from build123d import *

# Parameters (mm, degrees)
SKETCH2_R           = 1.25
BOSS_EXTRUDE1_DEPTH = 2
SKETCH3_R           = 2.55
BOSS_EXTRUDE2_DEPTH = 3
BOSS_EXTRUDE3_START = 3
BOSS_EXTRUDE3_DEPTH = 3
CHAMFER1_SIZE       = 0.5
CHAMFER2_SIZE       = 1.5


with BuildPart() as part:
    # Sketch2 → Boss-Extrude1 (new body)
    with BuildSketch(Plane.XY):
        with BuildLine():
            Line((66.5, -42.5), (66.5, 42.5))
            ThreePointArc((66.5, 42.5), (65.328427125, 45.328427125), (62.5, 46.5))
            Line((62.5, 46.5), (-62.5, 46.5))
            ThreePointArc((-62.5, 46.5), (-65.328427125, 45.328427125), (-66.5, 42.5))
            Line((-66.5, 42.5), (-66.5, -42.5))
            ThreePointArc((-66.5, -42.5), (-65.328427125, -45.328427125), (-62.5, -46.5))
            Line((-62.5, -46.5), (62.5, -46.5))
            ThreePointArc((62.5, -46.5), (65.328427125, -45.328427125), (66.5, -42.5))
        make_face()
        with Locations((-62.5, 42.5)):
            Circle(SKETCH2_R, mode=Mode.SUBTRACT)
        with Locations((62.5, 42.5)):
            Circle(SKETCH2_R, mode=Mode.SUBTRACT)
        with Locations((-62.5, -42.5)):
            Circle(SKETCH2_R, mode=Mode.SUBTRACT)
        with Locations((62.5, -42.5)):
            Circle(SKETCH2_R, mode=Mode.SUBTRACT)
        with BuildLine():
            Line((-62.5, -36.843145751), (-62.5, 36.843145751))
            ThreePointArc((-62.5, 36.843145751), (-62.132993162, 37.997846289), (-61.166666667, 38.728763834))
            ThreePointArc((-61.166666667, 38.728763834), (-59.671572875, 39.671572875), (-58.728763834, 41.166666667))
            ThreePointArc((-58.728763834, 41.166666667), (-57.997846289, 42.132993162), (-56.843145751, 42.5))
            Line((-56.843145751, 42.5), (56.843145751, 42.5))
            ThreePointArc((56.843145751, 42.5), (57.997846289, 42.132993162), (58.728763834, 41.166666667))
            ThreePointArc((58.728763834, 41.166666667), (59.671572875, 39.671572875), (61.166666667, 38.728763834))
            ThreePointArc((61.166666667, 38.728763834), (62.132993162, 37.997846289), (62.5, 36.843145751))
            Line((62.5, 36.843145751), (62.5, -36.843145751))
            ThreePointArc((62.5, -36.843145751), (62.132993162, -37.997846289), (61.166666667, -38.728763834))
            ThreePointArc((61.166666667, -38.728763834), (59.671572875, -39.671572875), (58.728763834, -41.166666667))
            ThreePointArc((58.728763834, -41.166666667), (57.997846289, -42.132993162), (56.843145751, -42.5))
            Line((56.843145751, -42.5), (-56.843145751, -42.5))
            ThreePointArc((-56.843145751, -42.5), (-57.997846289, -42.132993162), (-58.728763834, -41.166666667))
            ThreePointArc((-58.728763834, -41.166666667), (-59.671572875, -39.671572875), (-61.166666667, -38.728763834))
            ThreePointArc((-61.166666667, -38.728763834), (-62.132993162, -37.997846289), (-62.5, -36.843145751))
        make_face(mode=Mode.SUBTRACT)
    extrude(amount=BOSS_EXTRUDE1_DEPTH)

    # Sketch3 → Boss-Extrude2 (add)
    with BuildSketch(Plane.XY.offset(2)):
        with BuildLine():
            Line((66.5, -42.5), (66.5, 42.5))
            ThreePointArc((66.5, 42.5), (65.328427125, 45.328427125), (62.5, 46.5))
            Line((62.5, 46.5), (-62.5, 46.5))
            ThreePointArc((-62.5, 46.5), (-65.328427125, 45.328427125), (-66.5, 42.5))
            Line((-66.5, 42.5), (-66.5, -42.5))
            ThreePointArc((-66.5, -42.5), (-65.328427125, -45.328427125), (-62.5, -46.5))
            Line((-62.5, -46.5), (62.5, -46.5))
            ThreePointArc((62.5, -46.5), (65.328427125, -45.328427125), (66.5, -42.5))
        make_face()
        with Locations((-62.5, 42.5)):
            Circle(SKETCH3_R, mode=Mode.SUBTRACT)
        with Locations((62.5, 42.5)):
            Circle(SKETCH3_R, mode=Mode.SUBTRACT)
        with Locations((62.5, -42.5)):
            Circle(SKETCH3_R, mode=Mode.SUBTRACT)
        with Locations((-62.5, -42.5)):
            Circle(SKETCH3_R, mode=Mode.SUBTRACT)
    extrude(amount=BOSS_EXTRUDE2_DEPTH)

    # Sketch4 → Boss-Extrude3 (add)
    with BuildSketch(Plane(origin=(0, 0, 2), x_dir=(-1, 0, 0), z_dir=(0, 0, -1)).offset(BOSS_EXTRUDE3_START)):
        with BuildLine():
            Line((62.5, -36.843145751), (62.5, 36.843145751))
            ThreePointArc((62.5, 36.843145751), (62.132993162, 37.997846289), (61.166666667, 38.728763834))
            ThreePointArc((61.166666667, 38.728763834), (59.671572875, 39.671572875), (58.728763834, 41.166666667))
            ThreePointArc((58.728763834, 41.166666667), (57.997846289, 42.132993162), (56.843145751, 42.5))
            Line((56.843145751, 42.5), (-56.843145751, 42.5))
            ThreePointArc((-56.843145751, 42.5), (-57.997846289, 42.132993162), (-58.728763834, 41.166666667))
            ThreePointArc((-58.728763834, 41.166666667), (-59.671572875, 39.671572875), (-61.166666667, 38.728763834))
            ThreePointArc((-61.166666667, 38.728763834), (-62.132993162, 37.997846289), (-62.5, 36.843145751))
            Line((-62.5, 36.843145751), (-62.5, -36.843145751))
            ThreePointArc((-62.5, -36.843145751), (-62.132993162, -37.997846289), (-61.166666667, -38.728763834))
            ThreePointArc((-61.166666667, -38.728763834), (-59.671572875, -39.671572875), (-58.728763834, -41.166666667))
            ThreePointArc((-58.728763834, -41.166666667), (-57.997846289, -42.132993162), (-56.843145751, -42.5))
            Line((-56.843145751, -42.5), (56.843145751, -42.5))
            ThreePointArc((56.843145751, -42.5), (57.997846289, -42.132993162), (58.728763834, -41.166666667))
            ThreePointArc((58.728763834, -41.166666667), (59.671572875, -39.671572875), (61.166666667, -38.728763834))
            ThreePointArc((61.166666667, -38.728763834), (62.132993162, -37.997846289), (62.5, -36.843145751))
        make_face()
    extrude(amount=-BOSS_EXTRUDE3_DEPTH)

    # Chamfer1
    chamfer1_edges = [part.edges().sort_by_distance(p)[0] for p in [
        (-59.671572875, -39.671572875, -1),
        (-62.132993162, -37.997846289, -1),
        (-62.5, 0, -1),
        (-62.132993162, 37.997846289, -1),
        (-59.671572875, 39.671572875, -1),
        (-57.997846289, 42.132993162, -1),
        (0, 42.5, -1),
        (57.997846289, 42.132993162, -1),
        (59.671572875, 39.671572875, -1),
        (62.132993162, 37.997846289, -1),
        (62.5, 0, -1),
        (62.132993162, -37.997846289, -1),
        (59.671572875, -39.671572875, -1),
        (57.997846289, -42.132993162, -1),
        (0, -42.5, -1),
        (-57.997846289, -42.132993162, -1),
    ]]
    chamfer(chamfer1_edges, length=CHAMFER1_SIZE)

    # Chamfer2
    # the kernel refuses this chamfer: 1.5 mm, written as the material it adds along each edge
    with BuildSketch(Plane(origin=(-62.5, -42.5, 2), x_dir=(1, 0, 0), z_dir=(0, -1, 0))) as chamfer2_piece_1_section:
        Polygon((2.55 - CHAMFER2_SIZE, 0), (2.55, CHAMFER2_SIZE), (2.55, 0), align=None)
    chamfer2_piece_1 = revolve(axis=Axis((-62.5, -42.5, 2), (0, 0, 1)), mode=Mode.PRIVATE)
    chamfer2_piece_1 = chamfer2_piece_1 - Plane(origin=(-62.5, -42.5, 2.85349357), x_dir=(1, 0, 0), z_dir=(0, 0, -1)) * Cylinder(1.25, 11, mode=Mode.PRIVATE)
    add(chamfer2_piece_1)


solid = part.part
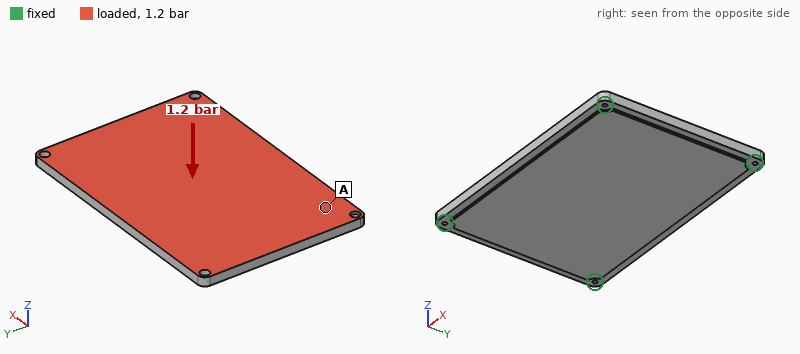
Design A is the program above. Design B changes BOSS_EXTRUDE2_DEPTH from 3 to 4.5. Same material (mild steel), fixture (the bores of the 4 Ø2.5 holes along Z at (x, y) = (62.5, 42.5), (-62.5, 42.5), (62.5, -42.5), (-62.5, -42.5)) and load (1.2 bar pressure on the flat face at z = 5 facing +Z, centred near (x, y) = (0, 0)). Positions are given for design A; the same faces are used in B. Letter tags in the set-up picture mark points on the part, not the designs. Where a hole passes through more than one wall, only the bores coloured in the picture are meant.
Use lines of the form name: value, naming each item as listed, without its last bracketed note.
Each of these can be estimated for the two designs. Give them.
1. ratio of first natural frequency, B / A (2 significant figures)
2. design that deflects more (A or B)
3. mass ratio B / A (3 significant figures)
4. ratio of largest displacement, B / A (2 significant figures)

ratio of first natural frequency, B / A: 1.2
design that deflects more: A
mass ratio B / A: 1.26
ratio of largest displacement, B / A: 0.54
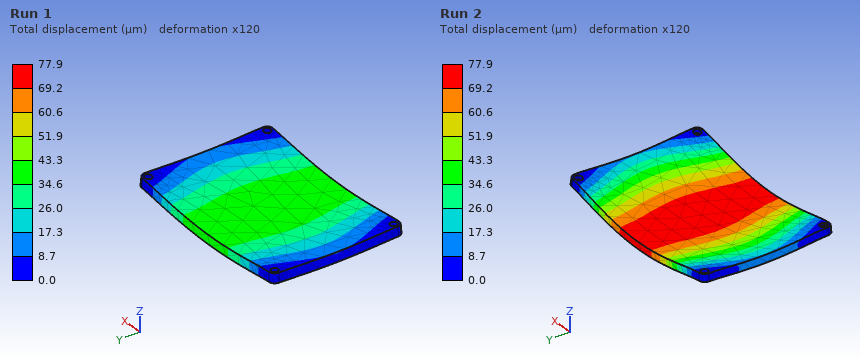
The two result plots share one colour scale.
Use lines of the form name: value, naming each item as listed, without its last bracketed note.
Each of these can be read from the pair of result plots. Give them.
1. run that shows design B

run that shows design B: Run 1
